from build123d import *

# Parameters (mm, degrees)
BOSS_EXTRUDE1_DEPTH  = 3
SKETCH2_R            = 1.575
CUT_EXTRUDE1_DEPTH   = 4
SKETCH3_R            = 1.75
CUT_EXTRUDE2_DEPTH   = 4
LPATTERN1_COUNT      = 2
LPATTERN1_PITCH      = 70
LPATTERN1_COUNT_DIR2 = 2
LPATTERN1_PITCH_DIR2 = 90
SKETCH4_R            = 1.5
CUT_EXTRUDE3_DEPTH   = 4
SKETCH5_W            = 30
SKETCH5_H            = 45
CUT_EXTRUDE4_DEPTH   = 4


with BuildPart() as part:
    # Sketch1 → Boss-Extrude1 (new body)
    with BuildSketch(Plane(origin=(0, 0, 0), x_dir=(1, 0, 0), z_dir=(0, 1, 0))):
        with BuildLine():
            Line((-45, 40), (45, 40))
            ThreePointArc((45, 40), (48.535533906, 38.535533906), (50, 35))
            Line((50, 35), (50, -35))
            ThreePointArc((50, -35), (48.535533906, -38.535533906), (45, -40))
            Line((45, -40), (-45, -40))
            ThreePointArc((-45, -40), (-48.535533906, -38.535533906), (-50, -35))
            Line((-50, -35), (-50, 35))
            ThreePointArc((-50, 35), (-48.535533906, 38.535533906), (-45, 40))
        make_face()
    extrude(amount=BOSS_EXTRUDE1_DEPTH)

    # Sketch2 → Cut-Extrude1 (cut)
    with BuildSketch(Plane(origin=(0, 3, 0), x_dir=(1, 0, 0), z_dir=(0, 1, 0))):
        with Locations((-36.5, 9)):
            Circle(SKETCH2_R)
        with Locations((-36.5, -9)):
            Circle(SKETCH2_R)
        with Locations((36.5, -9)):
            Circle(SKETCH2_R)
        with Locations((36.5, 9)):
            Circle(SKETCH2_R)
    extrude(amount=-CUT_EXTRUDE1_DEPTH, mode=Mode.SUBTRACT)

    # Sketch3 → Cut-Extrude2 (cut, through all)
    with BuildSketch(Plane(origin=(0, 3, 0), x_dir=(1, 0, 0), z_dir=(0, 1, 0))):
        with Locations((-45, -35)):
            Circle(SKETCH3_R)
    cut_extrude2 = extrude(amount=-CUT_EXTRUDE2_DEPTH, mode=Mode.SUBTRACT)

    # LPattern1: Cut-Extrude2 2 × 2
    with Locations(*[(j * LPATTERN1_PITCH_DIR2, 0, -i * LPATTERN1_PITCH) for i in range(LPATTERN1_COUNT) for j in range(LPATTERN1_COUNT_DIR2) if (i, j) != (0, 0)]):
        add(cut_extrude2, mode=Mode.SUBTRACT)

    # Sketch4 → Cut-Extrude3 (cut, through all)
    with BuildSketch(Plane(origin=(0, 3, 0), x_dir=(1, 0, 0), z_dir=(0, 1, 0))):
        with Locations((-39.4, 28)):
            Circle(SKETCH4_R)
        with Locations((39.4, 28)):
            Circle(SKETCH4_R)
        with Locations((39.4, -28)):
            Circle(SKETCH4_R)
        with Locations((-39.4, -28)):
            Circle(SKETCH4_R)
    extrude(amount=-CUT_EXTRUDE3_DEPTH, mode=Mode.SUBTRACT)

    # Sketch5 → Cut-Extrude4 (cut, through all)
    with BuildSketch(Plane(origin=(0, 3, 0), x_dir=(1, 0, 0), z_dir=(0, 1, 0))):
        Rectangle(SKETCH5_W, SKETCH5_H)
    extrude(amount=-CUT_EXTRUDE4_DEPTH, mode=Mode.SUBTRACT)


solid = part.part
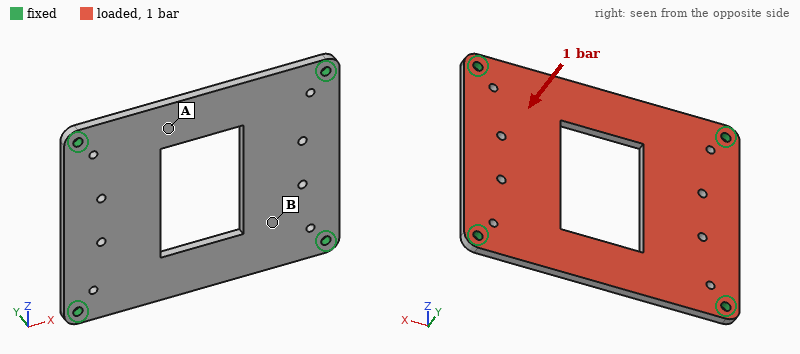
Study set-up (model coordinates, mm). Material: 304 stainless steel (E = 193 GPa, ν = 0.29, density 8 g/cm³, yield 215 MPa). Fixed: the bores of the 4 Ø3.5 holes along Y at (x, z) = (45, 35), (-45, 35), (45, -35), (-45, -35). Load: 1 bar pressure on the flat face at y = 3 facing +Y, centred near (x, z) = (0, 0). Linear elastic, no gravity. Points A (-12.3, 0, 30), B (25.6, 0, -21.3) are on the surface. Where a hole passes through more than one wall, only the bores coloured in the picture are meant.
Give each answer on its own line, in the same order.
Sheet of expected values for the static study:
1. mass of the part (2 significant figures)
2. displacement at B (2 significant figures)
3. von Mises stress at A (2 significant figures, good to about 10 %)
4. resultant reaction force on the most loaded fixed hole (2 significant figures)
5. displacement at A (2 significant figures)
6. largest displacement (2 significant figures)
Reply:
160 g
42 µm
26 MPa
160 N
55 µm
76 µm
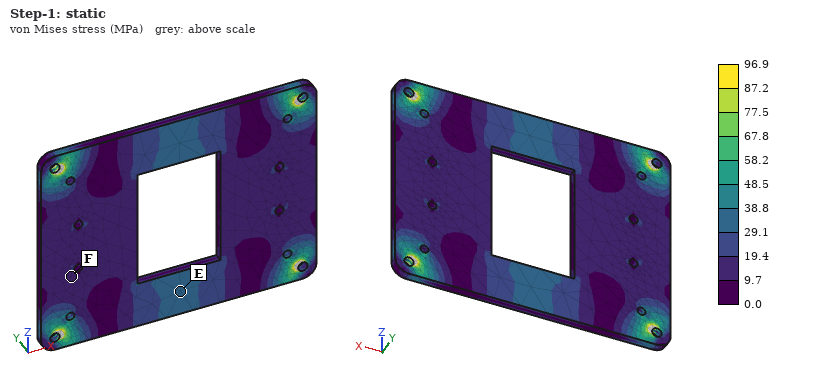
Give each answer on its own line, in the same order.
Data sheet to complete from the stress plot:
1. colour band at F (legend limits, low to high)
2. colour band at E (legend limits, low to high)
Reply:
9.7 to 19.4 MPa
29.1 to 38.8 MPa
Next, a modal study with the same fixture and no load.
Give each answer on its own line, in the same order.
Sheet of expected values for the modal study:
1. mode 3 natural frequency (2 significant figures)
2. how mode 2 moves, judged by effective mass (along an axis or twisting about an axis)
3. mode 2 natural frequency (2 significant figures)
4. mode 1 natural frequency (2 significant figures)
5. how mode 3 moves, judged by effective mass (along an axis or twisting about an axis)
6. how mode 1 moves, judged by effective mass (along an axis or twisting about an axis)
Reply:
2600 Hz
twisting about X
2200 Hz
1500 Hz
twisting about Z
along Y
